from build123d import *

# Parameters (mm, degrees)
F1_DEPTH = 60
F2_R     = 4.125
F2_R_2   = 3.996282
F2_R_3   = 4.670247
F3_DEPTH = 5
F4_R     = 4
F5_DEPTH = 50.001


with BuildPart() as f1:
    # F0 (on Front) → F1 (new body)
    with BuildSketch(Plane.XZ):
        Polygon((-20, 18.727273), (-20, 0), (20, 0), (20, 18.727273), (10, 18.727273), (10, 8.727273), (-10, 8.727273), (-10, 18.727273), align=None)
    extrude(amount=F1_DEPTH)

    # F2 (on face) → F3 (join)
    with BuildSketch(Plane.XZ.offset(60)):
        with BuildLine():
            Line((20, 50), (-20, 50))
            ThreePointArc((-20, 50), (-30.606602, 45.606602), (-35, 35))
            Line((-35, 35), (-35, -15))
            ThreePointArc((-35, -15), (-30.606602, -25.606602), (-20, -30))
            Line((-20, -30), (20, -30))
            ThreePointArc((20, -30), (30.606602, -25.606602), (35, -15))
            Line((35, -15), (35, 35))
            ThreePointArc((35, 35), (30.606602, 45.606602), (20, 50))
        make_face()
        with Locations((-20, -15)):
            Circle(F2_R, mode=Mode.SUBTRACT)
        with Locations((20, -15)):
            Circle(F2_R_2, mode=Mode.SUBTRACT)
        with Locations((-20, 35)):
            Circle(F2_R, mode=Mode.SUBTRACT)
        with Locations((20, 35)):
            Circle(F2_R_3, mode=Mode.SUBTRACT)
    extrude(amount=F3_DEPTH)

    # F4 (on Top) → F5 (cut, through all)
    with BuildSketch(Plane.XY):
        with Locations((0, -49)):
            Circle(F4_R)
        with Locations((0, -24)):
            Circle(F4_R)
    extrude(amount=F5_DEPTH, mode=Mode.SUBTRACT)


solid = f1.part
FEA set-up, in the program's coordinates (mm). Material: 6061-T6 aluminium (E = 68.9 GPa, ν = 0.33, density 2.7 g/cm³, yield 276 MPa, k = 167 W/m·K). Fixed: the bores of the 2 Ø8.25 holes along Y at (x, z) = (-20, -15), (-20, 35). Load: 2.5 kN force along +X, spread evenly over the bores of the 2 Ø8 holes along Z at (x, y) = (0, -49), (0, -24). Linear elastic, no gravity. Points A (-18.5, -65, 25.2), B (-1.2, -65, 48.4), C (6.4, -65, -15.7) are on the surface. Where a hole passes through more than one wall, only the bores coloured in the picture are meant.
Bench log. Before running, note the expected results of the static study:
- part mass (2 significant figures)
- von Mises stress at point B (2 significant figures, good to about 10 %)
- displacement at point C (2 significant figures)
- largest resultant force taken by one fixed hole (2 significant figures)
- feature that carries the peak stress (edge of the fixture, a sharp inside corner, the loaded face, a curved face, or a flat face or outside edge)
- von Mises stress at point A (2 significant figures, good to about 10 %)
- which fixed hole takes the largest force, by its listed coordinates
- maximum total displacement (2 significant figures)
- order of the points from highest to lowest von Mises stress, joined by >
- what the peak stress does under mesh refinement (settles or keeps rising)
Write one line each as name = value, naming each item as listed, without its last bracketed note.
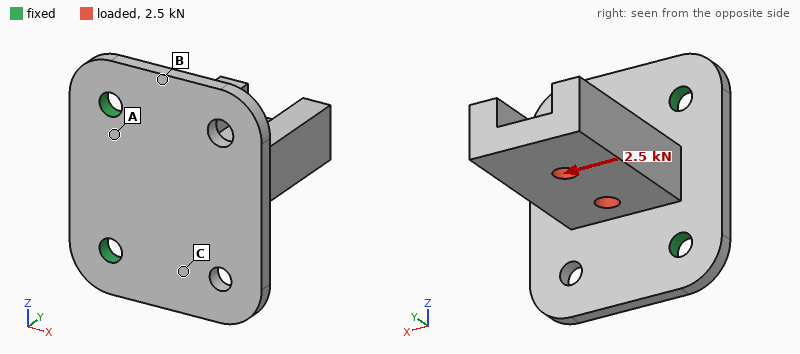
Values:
part mass = 160 g
von Mises stress at point B = 66 MPa
displacement at point C = 0.21 mm
largest resultant force taken by one fixed hole = 1.5 kN
feature that carries the peak stress = edge of the fixture
von Mises stress at point A = 120 MPa
which fixed hole takes the largest force, by its listed coordinates = (-20, -15)
maximum total displacement = 0.85 mm
order of the points from highest to lowest von Mises stress, joined by > = A > B > C
what the peak stress does under mesh refinement = keeps rising
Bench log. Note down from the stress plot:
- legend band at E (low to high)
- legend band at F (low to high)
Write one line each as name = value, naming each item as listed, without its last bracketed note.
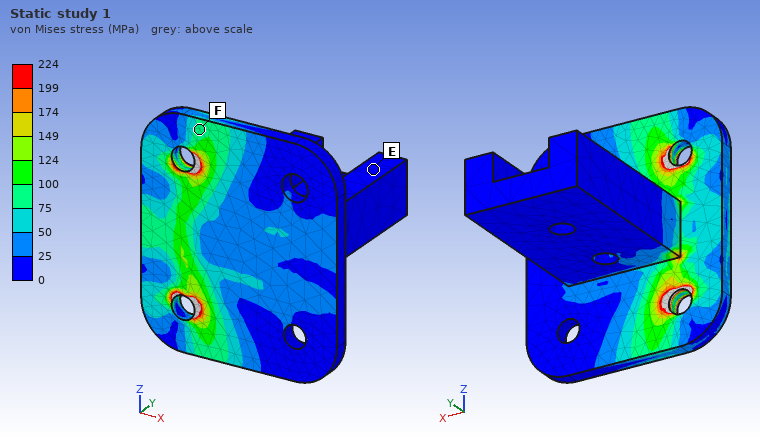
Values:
legend band at E = 0 to 25 MPa
legend band at F = 75 to 100 MPa
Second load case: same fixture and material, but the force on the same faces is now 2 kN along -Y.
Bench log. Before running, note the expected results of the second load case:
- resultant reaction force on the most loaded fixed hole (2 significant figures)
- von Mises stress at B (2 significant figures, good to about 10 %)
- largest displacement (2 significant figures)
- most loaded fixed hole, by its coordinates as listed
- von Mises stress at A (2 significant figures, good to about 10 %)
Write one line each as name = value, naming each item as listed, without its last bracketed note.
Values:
resultant reaction force on the most loaded fixed hole = 1.3 kN
von Mises stress at B = 37 MPa
largest displacement = 0.44 mm
most loaded fixed hole, by its coordinates as listed = (-20, -15)
von Mises stress at A = 68 MPa
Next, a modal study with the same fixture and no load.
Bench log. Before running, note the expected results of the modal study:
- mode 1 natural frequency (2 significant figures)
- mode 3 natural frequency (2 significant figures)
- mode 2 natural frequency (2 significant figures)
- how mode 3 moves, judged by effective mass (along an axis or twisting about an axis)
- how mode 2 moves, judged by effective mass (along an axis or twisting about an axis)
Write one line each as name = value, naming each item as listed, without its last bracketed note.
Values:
mode 1 natural frequency = 840 Hz
mode 3 natural frequency = 4000 Hz
mode 2 natural frequency = 1700 Hz
how mode 3 moves, judged by effective mass = along Y
how mode 2 moves, judged by effective mass = along Z
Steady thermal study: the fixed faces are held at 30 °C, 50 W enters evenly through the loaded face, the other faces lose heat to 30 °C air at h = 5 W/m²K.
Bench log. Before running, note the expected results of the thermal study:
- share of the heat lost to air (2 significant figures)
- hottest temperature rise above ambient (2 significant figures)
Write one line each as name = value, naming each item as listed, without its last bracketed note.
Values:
share of the heat lost to air = 3.7 %
hottest temperature rise above ambient = 35 K
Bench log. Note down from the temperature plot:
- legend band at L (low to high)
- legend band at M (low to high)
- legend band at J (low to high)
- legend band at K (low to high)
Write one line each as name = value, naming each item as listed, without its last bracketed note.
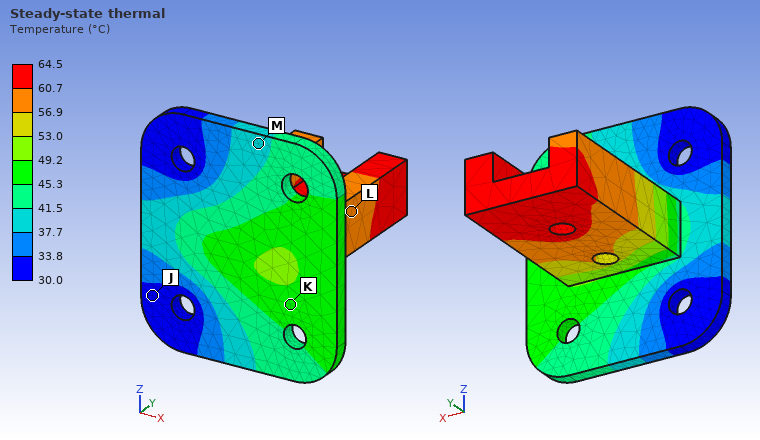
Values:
legend band at L = 56.9 to 60.7 °C
legend band at M = 37.7 to 41.5 °C
legend band at J = 30.0 to 33.8 °C
legend band at K = 45.3 to 49.2 °C
